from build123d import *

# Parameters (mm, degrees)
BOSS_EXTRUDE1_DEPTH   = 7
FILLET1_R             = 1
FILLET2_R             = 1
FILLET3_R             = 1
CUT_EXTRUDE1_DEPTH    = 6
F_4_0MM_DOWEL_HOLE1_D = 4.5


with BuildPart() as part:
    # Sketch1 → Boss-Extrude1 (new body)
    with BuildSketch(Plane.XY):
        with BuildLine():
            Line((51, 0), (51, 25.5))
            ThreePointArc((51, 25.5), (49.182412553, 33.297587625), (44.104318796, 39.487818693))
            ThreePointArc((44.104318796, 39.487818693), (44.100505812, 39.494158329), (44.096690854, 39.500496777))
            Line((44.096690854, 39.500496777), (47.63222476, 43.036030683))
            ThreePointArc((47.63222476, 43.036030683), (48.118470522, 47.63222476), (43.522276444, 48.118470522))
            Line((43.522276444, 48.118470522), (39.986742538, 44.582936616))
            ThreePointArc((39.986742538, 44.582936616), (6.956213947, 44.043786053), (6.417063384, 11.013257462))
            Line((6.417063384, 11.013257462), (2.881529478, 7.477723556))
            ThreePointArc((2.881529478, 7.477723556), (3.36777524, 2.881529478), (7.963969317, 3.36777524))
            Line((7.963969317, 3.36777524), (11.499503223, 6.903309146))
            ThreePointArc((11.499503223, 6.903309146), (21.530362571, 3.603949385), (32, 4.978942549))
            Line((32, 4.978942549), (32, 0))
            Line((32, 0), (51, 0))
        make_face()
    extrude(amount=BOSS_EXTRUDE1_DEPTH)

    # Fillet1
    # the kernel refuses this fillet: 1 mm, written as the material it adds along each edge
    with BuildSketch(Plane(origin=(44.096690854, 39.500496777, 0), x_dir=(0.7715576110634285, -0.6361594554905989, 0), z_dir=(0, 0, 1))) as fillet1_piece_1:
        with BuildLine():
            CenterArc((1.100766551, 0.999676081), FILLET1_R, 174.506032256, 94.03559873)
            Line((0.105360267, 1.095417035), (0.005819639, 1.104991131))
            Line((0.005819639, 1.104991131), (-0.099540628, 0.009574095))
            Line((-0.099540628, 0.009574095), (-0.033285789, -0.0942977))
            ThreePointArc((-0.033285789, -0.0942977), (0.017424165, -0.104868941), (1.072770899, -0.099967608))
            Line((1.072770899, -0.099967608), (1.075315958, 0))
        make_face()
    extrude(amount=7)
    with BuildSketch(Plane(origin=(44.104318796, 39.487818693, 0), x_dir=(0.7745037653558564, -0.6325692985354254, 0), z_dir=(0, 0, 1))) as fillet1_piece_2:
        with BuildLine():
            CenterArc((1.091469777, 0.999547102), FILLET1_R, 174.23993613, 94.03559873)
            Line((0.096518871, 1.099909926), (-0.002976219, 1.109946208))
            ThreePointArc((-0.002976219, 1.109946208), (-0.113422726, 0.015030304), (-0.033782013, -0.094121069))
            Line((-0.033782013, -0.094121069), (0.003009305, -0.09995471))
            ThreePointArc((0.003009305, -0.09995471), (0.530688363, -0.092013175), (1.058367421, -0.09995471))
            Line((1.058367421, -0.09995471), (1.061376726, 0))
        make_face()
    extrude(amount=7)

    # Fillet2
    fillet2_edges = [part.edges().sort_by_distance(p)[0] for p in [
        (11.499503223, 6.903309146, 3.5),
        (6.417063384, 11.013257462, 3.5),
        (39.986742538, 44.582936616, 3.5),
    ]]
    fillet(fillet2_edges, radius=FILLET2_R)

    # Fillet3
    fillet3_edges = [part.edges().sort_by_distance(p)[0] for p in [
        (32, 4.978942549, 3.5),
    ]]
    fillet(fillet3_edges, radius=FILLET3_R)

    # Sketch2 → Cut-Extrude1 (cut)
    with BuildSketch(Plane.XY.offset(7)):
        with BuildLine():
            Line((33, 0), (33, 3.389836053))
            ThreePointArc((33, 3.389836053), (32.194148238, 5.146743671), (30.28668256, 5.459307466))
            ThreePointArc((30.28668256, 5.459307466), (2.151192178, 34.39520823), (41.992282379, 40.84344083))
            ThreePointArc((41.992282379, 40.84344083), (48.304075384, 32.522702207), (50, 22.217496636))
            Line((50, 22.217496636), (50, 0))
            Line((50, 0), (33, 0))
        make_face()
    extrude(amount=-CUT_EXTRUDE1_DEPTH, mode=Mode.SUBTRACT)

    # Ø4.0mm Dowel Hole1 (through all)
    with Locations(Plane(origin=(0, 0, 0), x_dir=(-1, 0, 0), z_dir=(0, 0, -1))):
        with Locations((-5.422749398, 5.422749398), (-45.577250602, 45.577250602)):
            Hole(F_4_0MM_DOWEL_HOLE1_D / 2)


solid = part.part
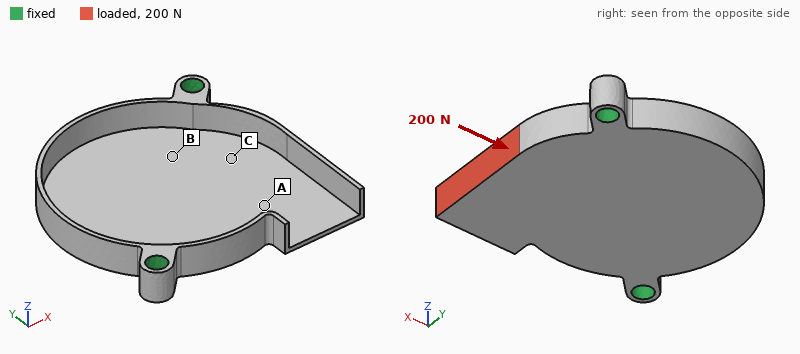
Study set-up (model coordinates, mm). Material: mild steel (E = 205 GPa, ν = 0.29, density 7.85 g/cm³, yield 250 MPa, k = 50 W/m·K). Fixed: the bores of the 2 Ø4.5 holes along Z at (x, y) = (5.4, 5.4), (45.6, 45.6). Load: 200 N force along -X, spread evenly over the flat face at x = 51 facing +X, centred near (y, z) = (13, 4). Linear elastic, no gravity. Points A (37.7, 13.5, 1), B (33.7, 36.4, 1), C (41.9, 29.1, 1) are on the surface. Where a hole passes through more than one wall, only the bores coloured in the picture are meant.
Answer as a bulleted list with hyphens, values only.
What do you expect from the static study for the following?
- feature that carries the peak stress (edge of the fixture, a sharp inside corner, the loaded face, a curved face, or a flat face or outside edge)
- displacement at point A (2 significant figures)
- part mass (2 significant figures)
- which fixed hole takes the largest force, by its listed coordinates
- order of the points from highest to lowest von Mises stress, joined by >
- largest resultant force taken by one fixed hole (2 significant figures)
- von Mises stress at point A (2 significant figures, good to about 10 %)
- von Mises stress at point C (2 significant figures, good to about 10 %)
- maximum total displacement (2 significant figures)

- a curved face
- 18 µm
- 27 g
- (5.4, 5.4)
- A > C > B
- 150 N
- 35 MPa
- 21 MPa
- 84 µm
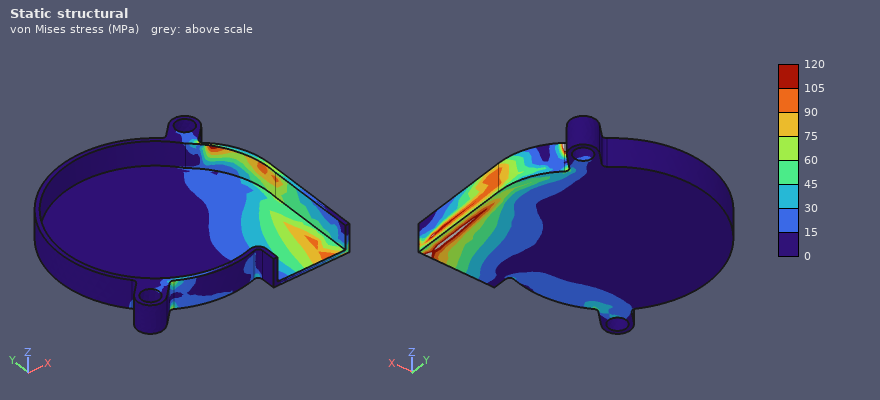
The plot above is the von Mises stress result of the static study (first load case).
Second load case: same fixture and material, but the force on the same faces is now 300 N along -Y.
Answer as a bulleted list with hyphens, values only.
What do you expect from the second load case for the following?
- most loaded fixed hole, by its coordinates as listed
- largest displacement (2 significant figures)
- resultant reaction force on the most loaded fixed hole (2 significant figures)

- (45.6, 45.6)
- 85 µm
- 300 N
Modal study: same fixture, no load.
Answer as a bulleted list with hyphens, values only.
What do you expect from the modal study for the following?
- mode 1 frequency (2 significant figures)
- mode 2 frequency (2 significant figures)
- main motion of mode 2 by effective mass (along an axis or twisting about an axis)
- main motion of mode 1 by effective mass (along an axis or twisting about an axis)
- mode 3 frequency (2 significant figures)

- 2200 Hz
- 3100 Hz
- along Z
- along Z
- 4100 Hz
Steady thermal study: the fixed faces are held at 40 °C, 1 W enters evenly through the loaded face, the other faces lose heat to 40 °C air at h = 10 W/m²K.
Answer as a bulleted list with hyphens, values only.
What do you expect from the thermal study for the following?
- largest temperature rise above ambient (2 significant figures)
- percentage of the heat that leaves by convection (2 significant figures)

- 18 K
- 26 %
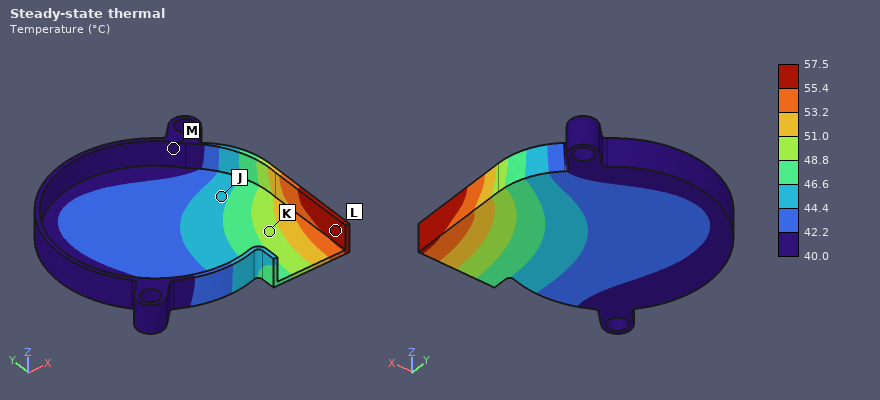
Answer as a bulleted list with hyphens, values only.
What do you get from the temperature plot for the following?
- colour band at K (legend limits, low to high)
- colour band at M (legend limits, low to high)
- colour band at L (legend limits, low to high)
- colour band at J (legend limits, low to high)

- 48.8 to 51.0 °C
- 40.0 to 42.2 °C
- 55.4 to 57.5 °C
- 44.4 to 46.6 °C
